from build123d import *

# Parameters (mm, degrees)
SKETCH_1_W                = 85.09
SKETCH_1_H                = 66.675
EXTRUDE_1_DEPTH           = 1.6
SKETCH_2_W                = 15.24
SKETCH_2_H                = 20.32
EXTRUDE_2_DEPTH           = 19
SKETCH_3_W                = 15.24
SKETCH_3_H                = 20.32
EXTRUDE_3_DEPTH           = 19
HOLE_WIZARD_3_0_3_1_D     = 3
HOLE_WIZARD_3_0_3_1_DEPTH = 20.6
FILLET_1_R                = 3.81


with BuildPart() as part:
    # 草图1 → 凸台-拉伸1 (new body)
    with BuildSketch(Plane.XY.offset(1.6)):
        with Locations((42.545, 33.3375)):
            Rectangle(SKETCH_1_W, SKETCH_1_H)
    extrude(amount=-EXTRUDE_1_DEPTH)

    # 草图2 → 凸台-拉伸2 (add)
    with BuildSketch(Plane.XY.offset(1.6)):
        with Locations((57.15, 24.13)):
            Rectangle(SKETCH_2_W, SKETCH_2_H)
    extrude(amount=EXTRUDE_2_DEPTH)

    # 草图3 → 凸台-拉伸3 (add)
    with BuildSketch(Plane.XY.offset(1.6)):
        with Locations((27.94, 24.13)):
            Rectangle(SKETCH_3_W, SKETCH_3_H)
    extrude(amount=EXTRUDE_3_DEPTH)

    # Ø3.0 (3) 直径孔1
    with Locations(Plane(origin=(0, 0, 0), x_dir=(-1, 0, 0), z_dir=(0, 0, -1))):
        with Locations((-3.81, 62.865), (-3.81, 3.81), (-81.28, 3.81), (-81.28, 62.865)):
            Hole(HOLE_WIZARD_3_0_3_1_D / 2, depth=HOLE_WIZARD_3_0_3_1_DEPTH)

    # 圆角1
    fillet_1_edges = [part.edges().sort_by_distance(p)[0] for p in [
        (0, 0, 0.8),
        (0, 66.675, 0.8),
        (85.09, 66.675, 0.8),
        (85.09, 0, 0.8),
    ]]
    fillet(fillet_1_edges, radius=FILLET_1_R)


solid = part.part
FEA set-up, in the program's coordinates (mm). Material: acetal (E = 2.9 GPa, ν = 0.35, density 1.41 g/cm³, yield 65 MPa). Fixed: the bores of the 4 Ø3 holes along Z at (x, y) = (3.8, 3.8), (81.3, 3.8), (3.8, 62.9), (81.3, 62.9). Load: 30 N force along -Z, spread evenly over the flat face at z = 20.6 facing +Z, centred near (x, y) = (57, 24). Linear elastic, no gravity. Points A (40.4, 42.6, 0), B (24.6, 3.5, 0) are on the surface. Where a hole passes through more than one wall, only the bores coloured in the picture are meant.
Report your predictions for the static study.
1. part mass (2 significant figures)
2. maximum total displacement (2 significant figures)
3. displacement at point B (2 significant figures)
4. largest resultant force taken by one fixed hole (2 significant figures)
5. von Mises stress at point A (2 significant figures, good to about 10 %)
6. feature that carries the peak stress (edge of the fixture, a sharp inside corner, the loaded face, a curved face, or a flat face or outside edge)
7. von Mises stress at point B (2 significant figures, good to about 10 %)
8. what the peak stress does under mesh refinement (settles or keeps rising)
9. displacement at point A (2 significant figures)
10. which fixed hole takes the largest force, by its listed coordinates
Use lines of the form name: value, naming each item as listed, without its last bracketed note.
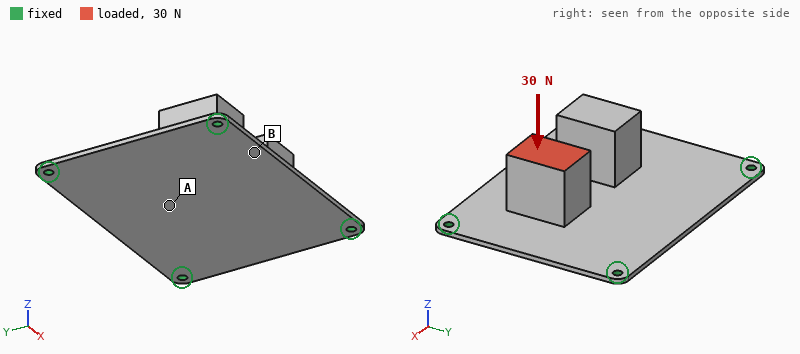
part mass: 29 g
maximum total displacement: 1.3 mm
displacement at point B: 0.56 mm
largest resultant force taken by one fixed hole: 15 N
von Mises stress at point A: 5.6 MPa
feature that carries the peak stress: edge of the fixture
von Mises stress at point B: 1.7 MPa
what the peak stress does under mesh refinement: keeps rising
displacement at point A: 1.0 mm
which fixed hole takes the largest force, by its listed coordinates: (81.3, 3.8)
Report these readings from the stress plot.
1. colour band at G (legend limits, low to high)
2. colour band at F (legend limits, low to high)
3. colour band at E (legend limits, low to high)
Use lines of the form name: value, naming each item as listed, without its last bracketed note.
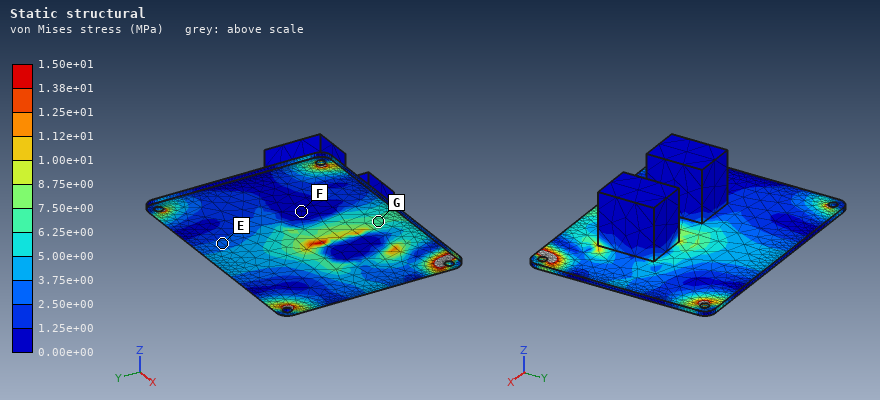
colour band at G: 6.25e+00 to 7.50e+00 MPa
colour band at F: 0.00e+00 to 1.25e+00 MPa
colour band at E: 2.50e+00 to 3.75e+00 MPa
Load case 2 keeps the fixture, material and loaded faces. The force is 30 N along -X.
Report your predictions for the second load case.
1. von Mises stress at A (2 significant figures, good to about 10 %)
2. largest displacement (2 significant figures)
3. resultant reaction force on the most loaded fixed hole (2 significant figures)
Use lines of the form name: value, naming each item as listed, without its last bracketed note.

von Mises stress at A: 6.0 MPa
largest displacement: 1.2 mm
resultant reaction force on the most loaded fixed hole: 13 N
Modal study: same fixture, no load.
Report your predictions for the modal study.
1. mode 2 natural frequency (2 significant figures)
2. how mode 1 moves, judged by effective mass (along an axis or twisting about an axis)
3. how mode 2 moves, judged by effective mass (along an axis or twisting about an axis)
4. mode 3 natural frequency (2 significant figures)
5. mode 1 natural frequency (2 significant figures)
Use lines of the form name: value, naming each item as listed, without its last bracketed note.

mode 2 natural frequency: 360 Hz
how mode 1 moves, judged by effective mass: along Z
how mode 2 moves, judged by effective mass: along Y
mode 3 natural frequency: 440 Hz
mode 1 natural frequency: 180 Hz
